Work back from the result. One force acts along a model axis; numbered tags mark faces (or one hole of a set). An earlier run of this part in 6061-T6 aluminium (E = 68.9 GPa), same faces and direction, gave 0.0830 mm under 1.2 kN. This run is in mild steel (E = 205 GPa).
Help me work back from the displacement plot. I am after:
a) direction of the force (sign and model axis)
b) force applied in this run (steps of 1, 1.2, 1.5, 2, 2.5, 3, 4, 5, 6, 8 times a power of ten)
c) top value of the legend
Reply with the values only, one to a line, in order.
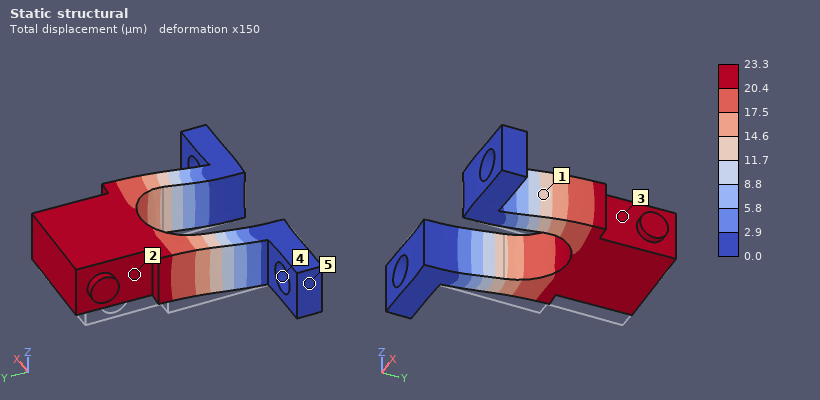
+X
1 kN
23.3 µm
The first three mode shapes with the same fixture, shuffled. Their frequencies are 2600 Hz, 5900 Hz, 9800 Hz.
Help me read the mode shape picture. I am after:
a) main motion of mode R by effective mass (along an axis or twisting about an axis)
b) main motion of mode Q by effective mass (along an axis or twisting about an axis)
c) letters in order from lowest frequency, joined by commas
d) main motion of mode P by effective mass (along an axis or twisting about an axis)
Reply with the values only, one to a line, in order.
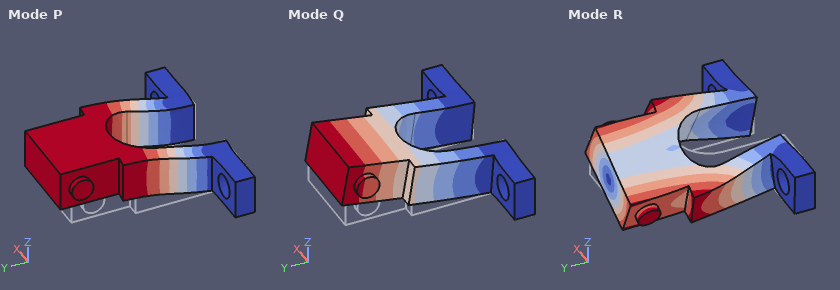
twisting about Y
along Z
Q, P, R
along X
